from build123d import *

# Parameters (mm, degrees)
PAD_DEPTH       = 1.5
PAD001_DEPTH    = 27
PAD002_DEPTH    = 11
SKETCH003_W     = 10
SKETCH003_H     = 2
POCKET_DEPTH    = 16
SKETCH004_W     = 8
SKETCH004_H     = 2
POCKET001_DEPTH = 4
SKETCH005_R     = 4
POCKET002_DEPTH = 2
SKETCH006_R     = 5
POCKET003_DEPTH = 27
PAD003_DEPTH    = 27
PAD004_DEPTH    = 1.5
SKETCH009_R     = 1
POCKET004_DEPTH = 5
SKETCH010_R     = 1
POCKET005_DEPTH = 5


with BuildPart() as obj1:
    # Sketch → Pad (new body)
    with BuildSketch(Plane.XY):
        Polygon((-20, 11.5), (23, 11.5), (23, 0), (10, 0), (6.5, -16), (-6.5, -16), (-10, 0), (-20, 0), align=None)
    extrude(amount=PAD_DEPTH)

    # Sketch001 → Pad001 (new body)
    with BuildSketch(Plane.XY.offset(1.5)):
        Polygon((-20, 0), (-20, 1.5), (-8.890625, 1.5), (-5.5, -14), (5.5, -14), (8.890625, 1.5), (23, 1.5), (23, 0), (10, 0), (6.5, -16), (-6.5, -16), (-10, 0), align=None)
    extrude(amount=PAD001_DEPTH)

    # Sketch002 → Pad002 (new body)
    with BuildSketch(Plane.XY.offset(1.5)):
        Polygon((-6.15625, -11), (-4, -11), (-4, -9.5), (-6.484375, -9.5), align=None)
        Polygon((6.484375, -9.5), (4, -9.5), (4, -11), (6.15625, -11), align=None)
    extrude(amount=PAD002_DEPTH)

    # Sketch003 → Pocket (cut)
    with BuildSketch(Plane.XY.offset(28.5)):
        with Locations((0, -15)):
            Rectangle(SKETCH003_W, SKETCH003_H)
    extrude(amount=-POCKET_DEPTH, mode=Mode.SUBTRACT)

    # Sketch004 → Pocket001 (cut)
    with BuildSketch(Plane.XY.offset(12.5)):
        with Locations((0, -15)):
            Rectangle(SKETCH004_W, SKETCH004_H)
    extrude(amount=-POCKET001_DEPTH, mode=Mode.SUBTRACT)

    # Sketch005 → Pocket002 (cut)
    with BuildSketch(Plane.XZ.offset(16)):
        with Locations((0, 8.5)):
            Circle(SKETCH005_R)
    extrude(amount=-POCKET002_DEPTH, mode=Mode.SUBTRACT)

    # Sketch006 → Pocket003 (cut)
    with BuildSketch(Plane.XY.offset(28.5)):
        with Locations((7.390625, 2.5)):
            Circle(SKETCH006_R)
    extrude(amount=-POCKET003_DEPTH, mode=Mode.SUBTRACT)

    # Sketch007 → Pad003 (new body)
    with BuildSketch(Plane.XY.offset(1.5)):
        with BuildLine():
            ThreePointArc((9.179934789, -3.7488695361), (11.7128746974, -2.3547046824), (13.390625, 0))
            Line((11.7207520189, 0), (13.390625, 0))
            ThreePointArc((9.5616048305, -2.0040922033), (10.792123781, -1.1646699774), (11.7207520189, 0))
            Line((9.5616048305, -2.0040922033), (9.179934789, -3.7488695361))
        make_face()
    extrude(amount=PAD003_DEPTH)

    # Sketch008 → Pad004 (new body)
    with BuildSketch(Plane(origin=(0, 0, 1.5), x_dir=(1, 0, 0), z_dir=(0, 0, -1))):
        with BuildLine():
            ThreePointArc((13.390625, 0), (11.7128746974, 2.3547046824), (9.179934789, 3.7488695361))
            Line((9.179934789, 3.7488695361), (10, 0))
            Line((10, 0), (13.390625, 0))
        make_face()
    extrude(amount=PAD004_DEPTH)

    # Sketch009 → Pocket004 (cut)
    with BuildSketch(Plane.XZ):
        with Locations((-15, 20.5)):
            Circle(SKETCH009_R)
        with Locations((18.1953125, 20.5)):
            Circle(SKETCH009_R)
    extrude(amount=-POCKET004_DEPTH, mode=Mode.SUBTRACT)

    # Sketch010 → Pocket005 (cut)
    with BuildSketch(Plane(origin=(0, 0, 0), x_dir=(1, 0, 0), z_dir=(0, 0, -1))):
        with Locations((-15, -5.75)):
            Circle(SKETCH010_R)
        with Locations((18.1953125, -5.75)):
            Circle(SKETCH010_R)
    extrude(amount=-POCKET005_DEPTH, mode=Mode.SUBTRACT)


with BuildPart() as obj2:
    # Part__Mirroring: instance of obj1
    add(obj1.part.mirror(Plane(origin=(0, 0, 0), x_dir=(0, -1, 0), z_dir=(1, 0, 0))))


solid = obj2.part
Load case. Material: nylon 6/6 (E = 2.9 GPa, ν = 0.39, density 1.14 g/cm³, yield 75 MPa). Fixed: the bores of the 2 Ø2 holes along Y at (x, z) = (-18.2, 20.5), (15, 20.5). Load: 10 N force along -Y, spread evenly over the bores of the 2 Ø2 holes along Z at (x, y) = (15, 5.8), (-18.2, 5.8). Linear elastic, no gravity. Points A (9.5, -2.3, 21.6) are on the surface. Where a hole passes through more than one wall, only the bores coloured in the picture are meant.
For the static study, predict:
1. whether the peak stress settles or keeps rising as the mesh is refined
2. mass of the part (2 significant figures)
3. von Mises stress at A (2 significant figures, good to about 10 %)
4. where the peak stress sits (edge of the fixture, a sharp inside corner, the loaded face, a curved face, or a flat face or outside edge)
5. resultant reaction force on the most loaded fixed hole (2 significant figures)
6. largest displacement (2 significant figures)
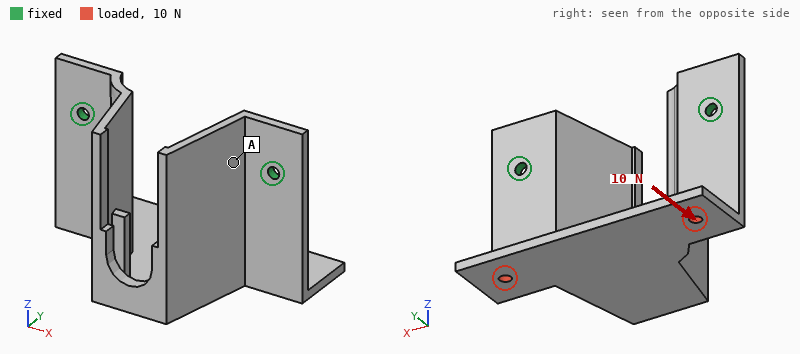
keeps rising
4.1 g
2.4 MPa
edge of the fixture
5.1 N
0.61 mm
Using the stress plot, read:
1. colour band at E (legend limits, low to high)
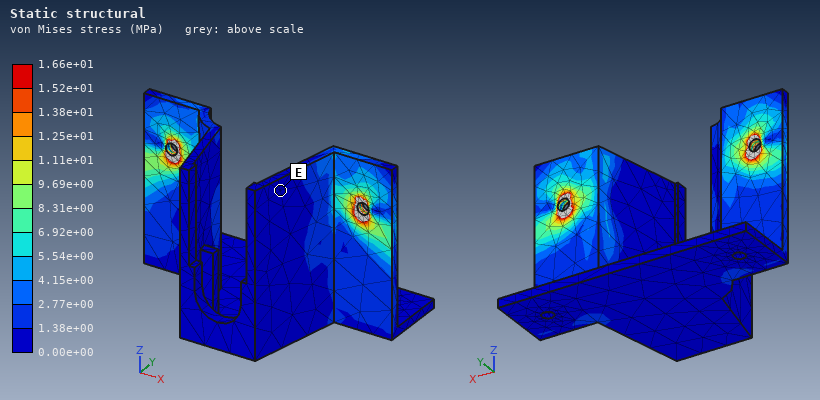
0.00e+00 to 1.38e+00 MPa
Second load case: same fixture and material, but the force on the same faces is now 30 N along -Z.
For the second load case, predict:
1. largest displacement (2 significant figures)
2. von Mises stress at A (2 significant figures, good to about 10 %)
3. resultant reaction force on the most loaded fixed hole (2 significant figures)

0.69 mm
2.4 MPa
15 N
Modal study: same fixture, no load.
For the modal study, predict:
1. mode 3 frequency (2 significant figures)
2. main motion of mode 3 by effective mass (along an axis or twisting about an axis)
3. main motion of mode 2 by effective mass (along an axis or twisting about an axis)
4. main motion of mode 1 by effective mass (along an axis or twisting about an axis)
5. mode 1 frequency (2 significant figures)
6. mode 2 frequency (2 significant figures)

1200 Hz
along X
twisting about Z
along Y
460 Hz
1000 Hz
